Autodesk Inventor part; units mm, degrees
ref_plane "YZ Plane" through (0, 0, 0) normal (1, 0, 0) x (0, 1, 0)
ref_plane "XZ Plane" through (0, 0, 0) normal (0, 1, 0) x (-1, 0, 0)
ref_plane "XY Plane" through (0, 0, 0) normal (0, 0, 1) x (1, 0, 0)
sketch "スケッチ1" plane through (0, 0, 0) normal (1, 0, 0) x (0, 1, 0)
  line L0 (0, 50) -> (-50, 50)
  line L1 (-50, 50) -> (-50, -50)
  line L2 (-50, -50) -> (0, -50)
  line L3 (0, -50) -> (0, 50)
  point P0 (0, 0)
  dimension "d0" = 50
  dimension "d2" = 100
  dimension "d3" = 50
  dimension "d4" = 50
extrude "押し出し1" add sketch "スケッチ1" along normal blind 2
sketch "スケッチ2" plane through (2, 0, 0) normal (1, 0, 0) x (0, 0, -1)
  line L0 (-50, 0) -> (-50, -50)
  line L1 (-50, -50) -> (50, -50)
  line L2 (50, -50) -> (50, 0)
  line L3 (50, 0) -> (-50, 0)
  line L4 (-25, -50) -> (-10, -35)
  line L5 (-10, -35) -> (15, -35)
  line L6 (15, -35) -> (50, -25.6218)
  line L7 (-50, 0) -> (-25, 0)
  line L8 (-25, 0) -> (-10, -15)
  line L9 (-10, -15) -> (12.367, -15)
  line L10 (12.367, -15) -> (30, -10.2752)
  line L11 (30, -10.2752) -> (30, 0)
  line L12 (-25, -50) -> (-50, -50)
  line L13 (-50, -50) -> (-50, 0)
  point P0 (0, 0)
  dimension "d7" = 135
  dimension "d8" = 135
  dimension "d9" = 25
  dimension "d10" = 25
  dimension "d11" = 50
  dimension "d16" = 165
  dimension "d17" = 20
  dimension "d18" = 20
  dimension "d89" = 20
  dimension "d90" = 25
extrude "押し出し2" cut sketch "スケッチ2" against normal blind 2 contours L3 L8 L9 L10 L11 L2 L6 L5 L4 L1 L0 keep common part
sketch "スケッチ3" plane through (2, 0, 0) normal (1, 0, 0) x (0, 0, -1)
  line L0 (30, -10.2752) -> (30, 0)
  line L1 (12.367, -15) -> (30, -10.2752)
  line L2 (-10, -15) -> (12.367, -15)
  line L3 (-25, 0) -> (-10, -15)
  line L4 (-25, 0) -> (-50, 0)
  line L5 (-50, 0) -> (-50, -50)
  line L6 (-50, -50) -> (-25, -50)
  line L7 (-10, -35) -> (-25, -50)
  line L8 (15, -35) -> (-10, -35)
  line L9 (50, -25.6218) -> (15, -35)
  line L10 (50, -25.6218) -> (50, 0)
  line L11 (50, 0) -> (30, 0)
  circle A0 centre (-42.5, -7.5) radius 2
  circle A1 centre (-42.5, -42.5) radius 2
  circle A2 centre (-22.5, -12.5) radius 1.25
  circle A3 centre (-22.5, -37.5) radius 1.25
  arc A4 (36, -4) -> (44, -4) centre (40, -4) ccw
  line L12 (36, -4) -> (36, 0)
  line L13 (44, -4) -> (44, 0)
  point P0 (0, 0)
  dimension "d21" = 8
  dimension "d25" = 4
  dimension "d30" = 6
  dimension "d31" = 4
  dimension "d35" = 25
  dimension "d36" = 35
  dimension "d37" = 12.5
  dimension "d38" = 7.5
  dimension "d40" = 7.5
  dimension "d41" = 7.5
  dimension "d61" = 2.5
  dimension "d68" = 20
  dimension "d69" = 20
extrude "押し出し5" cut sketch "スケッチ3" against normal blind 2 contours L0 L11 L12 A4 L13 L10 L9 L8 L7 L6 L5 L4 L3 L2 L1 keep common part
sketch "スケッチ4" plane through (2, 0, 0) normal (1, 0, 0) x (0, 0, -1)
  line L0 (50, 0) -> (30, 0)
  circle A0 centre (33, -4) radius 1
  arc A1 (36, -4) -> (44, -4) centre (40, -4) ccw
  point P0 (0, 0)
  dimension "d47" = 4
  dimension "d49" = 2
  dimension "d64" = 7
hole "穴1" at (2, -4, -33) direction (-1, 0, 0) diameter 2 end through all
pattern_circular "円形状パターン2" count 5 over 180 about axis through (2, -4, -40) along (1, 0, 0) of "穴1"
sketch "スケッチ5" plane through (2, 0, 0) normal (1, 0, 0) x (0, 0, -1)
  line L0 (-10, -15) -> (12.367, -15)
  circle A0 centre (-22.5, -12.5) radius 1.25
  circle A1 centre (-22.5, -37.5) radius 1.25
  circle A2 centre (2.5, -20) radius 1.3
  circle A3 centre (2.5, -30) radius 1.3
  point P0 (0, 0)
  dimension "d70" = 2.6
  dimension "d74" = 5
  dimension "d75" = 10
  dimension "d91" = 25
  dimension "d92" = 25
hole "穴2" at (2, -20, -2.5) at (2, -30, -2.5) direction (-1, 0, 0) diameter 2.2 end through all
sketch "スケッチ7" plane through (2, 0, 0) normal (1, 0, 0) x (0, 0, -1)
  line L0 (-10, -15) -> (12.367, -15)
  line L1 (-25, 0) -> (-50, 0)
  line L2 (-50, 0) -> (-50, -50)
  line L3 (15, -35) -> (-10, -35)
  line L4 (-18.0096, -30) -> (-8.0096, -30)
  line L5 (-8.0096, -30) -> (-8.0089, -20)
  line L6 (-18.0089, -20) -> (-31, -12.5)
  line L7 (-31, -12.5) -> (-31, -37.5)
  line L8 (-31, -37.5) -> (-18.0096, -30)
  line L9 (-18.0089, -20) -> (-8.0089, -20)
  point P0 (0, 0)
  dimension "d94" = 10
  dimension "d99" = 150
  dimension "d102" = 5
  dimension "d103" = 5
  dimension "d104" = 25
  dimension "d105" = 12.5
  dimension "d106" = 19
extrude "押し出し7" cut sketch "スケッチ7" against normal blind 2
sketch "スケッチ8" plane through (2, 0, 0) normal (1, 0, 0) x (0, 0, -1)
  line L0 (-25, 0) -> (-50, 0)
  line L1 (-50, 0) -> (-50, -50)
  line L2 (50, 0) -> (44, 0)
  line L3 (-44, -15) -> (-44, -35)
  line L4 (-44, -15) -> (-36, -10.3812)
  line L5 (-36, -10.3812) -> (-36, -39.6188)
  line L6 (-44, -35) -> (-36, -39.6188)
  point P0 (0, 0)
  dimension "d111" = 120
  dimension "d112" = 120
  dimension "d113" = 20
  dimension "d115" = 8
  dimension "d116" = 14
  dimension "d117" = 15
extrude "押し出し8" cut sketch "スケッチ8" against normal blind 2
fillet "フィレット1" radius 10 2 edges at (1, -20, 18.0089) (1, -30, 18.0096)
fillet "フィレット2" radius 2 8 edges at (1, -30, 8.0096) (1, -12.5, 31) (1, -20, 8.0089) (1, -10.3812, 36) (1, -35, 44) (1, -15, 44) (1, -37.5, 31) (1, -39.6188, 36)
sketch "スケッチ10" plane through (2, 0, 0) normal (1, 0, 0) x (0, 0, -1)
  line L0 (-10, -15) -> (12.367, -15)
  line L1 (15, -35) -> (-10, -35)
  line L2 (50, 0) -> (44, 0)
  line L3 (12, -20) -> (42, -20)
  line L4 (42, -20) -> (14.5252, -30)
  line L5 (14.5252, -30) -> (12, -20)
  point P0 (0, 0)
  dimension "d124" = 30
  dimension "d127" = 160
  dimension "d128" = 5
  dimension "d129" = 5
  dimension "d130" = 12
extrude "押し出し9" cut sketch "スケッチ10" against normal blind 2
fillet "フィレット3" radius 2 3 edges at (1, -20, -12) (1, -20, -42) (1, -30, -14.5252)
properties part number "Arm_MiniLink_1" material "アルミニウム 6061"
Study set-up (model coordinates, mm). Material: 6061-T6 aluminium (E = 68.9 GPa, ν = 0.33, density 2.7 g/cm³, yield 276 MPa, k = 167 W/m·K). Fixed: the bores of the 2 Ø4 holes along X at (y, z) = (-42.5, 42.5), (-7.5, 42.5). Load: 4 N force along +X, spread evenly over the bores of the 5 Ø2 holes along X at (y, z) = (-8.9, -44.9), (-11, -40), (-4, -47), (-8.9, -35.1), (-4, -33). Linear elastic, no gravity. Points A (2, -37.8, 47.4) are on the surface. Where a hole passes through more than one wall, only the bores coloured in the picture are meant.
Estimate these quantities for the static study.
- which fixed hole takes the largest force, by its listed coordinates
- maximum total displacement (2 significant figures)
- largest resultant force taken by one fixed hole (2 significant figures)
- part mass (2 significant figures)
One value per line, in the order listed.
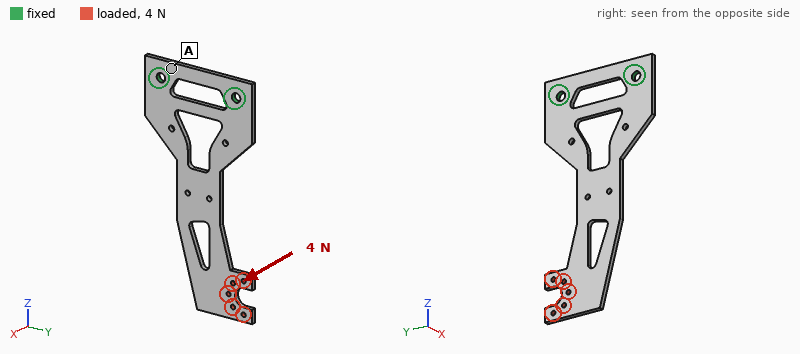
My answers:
(-7.5, 42.5)
1.1 mm
3.6 N
13 g
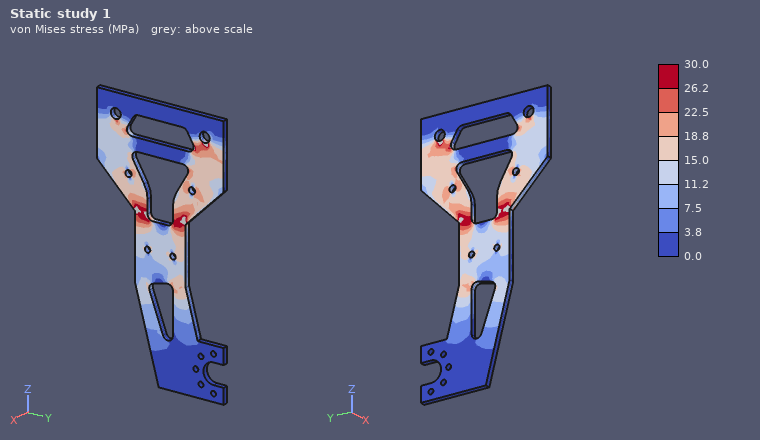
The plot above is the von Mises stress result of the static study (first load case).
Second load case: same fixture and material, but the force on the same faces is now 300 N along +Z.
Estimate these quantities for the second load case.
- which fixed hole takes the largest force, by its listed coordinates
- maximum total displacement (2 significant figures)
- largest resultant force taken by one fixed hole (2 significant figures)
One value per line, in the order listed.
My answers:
(-7.5, 42.5)
0.26 mm
350 N
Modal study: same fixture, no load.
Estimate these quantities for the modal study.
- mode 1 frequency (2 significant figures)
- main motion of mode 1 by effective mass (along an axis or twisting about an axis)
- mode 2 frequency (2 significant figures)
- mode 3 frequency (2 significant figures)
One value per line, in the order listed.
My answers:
190 Hz
along X
1000 Hz
1400 Hz
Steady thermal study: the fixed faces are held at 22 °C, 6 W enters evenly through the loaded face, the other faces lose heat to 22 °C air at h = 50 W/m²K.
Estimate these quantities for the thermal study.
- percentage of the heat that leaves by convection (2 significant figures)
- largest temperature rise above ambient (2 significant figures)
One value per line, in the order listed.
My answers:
71 %
47 K
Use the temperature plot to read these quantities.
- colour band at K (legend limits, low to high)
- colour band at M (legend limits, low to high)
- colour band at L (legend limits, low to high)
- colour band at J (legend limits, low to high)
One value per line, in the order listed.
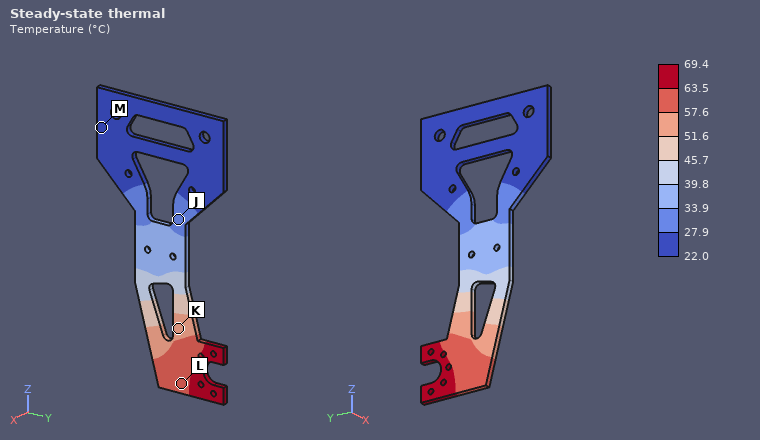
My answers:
51.6 to 57.6 °C
22.0 to 27.9 °C
57.6 to 63.5 °C
27.9 to 33.9 °C
